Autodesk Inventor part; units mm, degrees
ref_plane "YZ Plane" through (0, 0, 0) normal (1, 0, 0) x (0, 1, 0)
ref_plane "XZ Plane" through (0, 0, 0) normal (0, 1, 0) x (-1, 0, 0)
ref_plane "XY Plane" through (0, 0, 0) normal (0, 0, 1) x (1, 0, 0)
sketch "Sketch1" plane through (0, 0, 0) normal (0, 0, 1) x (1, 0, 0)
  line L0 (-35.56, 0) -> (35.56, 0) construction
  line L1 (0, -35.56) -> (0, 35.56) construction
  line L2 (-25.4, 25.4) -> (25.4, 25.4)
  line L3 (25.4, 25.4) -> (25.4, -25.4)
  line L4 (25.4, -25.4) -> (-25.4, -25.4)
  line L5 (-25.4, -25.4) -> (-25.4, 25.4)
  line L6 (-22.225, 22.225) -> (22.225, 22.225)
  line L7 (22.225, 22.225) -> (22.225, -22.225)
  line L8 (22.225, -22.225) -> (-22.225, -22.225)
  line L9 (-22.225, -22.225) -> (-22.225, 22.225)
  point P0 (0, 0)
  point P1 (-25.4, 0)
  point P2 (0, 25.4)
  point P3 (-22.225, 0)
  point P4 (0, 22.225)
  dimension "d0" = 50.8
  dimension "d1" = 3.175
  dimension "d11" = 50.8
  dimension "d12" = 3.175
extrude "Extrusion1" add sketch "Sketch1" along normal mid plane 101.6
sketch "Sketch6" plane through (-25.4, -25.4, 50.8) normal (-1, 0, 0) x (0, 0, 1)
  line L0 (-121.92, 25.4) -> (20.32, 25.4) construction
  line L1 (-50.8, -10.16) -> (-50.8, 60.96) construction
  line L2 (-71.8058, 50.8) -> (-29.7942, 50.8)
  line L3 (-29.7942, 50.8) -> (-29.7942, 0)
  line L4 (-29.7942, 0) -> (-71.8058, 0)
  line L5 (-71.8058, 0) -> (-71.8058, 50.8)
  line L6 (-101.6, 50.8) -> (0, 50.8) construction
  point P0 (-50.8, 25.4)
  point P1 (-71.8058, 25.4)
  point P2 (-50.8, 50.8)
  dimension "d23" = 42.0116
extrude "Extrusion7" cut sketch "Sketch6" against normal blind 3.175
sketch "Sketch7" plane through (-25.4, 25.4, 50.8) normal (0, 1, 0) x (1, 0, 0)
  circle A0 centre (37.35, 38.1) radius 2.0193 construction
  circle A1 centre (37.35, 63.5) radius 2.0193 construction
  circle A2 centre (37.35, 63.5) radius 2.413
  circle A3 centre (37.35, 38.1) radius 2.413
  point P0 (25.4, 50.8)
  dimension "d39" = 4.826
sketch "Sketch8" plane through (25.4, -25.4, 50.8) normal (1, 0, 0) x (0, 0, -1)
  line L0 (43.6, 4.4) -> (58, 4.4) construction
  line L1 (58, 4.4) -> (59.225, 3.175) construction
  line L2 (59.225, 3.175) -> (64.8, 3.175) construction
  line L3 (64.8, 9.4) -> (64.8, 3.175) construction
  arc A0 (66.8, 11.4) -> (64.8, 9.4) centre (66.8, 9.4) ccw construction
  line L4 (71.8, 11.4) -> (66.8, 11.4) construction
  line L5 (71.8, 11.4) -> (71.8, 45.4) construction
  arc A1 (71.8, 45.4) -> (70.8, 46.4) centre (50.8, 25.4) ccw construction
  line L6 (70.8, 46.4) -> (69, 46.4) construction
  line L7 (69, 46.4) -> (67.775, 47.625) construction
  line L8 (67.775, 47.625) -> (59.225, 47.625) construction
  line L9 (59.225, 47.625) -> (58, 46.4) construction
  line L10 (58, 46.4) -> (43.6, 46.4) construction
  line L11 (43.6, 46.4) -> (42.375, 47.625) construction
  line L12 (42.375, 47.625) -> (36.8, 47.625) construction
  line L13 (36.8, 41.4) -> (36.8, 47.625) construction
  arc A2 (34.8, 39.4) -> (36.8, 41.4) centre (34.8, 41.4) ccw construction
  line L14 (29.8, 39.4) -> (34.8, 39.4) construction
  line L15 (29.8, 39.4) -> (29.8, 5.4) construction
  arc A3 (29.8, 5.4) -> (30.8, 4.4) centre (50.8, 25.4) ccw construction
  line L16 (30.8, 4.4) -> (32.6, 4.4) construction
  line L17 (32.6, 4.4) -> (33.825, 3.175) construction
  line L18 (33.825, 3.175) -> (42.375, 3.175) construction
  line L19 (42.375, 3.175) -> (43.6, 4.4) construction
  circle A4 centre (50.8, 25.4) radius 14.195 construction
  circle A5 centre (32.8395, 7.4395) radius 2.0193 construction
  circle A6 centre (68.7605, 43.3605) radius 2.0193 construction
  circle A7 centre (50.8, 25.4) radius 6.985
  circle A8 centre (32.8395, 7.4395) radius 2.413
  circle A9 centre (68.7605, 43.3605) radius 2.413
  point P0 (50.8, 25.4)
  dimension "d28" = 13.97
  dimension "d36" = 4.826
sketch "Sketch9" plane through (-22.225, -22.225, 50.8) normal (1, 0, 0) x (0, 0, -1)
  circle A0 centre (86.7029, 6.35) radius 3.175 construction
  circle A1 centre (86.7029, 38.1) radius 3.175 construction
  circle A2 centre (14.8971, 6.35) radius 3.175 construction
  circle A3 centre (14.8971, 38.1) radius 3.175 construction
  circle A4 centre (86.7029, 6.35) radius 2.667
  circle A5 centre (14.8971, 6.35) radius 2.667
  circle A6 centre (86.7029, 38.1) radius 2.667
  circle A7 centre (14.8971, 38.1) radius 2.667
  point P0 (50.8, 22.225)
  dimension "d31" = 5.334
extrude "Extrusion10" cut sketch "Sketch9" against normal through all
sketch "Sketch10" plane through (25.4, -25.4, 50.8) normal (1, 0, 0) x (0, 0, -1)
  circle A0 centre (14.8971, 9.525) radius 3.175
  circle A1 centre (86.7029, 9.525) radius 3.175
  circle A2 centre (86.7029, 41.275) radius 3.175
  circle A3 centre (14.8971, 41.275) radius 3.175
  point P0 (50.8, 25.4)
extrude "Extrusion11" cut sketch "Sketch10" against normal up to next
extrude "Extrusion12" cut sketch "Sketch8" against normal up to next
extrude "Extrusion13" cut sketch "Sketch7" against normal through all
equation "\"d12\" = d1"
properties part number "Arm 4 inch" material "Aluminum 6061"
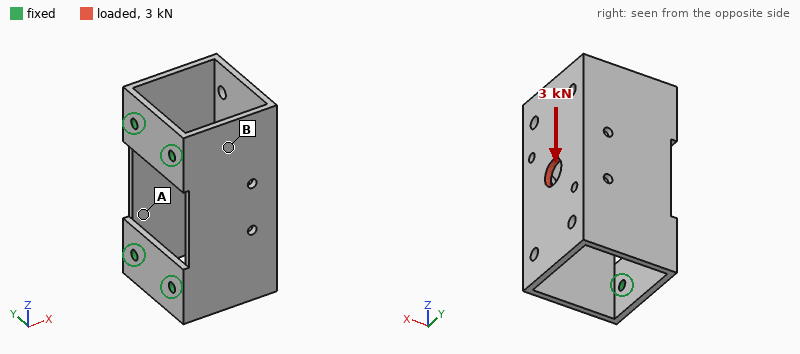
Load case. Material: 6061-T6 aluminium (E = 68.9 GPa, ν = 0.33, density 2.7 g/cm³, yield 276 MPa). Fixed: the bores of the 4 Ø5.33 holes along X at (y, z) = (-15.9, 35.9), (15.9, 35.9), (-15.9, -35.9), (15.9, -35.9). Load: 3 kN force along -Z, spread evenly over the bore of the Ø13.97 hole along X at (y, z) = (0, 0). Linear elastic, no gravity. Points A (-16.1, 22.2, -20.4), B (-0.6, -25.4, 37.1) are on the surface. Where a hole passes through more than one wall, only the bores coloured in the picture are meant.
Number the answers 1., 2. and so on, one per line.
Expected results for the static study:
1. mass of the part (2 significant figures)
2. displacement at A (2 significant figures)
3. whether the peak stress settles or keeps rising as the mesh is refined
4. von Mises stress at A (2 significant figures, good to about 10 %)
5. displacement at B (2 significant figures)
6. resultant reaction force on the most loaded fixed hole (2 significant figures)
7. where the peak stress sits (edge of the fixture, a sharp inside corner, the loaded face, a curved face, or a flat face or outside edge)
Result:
1. 140 g
2. 21 µm
3. keeps rising
4. 27 MPa
5. 43 µm
6. 1.2 kN
7. edge of the fixture
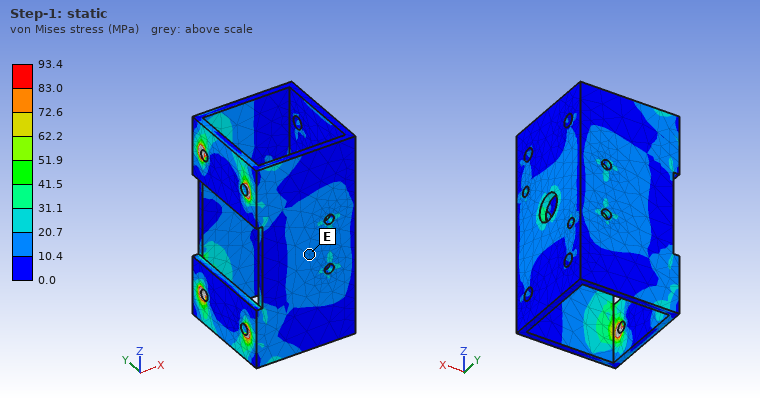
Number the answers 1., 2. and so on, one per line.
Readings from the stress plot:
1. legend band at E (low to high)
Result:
1. 10.4 to 20.7 MPa
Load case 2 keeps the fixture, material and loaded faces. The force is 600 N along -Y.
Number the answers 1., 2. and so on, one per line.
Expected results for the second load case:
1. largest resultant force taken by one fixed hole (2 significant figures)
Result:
1. 270 N
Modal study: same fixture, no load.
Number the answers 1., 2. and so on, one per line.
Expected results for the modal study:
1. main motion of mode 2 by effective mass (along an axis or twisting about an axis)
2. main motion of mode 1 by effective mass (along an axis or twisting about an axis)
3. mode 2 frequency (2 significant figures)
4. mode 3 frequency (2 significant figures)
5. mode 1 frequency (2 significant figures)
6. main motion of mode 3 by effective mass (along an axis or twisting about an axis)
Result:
1. along X
2. along Y
3. 3200 Hz
4. 3400 Hz
5. 770 Hz
6. along Z
